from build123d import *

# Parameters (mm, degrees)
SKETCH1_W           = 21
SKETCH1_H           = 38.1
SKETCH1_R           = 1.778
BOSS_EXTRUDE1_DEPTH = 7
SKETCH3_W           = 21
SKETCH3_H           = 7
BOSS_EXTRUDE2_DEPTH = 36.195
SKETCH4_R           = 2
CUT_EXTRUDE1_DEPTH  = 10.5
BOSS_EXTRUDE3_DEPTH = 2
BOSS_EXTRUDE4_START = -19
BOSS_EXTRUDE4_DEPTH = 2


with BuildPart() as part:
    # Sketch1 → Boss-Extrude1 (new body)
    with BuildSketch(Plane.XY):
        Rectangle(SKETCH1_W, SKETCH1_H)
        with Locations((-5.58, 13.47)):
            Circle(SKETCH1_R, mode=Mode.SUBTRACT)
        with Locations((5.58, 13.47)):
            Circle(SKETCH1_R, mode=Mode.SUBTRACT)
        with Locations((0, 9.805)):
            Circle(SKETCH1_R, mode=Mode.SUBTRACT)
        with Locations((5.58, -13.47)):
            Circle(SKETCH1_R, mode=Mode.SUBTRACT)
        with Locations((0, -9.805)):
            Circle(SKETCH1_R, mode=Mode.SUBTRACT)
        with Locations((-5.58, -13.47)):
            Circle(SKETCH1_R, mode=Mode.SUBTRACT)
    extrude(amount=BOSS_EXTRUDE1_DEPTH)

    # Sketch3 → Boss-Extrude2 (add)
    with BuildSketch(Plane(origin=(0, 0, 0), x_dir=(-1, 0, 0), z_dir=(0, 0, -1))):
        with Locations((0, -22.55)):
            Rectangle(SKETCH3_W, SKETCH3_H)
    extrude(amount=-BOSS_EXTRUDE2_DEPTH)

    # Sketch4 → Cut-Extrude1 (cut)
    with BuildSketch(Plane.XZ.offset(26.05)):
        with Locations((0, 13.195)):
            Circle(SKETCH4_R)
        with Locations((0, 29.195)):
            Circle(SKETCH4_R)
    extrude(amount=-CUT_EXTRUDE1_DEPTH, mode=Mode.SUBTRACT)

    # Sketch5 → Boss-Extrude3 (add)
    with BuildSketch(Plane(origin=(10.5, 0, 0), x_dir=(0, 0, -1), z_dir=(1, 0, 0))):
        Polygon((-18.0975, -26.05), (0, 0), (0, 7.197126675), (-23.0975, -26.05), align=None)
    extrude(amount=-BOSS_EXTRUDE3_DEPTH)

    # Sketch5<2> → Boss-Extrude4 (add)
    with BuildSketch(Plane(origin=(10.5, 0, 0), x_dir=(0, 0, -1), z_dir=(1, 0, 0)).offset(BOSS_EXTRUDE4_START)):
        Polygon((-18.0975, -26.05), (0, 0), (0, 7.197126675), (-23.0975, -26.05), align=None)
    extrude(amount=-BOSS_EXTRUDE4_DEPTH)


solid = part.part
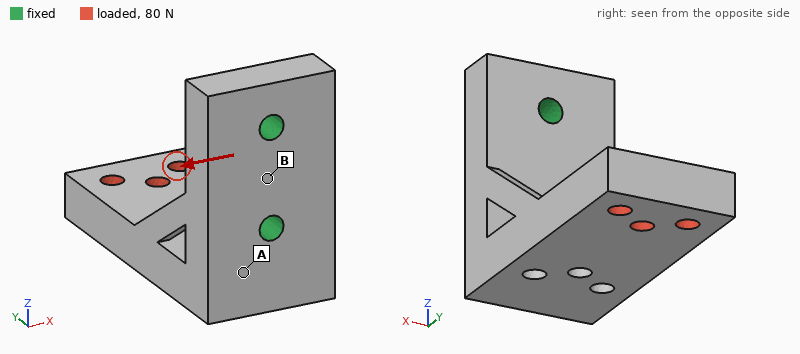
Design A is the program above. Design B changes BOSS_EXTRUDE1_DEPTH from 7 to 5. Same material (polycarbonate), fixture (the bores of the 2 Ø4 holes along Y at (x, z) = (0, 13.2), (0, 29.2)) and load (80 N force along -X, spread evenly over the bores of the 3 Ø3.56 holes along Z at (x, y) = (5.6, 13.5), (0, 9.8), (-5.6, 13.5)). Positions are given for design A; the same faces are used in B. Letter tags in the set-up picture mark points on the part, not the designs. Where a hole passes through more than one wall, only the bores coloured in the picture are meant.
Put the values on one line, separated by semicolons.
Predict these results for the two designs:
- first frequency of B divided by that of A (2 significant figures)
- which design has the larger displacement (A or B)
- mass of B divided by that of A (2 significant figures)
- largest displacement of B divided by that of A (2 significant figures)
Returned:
1.1; B; 0.87; 1.3
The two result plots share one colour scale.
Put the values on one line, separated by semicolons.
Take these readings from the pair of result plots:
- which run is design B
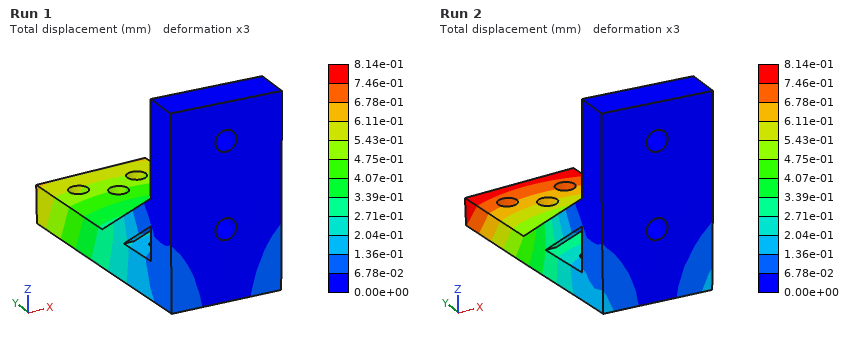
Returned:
Run 2
